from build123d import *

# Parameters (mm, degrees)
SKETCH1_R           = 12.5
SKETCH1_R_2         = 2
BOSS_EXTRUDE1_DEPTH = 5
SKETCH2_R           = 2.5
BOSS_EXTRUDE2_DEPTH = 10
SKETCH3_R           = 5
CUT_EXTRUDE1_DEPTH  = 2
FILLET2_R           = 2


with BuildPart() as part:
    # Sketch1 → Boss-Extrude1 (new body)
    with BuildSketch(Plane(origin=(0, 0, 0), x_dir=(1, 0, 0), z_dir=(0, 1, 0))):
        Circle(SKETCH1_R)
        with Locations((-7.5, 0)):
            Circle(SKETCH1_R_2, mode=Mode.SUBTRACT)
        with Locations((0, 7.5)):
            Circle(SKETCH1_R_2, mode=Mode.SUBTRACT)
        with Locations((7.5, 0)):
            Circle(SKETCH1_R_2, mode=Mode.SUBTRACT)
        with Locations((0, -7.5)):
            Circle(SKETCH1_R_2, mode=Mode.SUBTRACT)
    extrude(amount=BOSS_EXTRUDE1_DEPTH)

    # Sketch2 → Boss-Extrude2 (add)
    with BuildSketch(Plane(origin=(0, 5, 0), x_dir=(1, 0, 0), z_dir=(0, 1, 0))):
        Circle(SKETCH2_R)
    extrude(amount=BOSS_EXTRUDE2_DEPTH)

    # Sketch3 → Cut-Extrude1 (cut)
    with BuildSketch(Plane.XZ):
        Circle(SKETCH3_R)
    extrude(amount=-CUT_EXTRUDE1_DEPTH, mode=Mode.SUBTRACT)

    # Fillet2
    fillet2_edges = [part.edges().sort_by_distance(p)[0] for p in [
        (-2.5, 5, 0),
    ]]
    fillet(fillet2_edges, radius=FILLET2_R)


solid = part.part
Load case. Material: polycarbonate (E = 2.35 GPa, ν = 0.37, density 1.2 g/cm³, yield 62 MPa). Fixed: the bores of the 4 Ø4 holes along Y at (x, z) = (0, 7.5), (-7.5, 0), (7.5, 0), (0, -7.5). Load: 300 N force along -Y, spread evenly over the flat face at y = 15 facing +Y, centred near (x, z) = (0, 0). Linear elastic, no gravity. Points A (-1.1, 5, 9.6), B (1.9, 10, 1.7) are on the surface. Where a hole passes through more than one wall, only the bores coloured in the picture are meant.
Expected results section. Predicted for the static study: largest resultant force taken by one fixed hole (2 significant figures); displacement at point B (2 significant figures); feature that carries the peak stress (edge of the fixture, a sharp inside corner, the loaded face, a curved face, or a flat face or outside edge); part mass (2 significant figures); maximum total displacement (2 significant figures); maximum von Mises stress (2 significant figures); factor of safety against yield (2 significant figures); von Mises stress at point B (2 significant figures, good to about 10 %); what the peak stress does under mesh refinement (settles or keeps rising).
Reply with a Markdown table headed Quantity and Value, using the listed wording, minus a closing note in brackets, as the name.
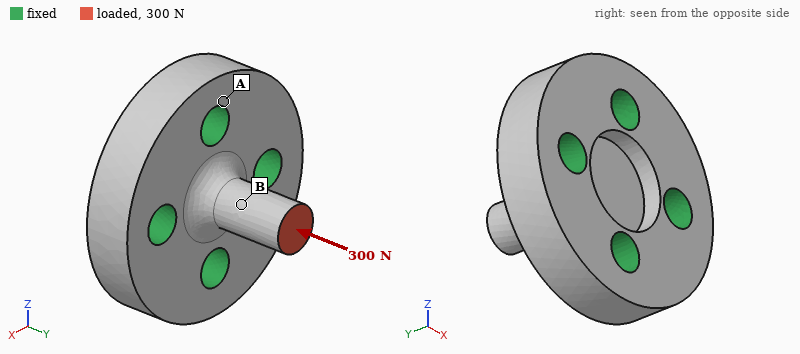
| Quantity | Value |
|---|---|
| largest resultant force taken by one fixed hole | 87 N |
| displacement at point B | 52 µm |
| feature that carries the peak stress | a curved face |
| part mass | 2.7 g |
| maximum total displacement | 85 µm |
| maximum von Mises stress | 21 MPa |
| factor of safety against yield | 3.0 |
| von Mises stress at point B | 15 MPa |
| what the peak stress does under mesh refinement | settles |
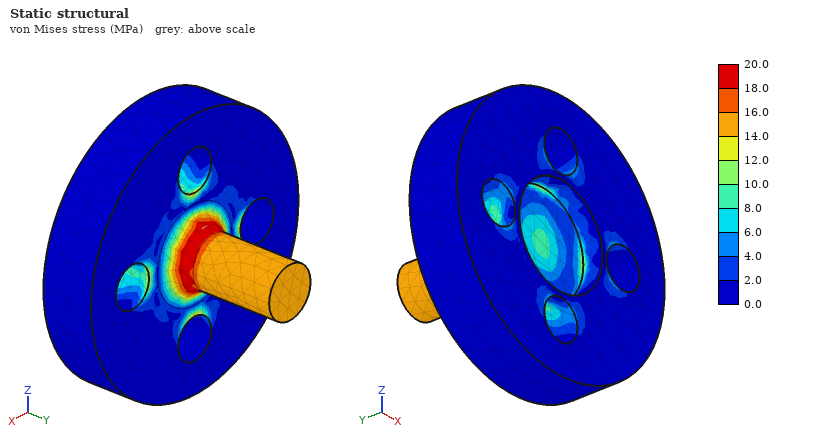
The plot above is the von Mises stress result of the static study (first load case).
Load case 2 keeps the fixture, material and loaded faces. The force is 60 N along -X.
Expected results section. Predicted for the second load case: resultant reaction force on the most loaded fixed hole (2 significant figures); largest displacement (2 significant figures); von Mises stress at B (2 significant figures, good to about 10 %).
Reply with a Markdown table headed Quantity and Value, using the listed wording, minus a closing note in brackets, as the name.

| Quantity | Value |
|---|---|
| resultant reaction force on the most loaded fixed hole | 65 N |
| largest displacement | 0.34 mm |
| von Mises stress at B | 19 MPa |
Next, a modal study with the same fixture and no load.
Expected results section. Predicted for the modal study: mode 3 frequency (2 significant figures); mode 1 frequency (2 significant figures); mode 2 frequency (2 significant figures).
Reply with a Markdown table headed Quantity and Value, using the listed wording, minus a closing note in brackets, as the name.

| Quantity | Value |
|---|---|
| mode 3 frequency | 22 kHz |
| mode 1 frequency | 8600 Hz |
| mode 2 frequency | 8600 Hz |
